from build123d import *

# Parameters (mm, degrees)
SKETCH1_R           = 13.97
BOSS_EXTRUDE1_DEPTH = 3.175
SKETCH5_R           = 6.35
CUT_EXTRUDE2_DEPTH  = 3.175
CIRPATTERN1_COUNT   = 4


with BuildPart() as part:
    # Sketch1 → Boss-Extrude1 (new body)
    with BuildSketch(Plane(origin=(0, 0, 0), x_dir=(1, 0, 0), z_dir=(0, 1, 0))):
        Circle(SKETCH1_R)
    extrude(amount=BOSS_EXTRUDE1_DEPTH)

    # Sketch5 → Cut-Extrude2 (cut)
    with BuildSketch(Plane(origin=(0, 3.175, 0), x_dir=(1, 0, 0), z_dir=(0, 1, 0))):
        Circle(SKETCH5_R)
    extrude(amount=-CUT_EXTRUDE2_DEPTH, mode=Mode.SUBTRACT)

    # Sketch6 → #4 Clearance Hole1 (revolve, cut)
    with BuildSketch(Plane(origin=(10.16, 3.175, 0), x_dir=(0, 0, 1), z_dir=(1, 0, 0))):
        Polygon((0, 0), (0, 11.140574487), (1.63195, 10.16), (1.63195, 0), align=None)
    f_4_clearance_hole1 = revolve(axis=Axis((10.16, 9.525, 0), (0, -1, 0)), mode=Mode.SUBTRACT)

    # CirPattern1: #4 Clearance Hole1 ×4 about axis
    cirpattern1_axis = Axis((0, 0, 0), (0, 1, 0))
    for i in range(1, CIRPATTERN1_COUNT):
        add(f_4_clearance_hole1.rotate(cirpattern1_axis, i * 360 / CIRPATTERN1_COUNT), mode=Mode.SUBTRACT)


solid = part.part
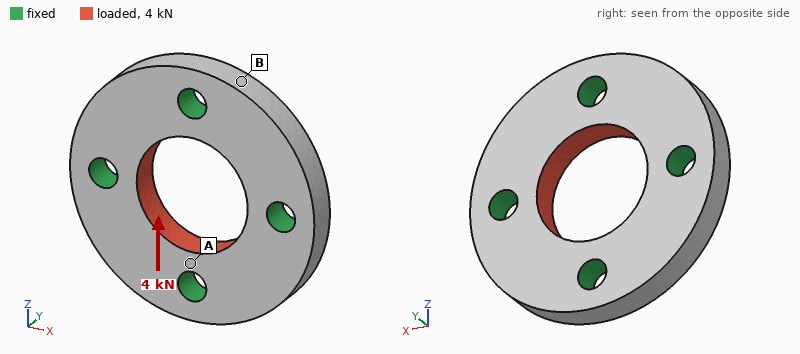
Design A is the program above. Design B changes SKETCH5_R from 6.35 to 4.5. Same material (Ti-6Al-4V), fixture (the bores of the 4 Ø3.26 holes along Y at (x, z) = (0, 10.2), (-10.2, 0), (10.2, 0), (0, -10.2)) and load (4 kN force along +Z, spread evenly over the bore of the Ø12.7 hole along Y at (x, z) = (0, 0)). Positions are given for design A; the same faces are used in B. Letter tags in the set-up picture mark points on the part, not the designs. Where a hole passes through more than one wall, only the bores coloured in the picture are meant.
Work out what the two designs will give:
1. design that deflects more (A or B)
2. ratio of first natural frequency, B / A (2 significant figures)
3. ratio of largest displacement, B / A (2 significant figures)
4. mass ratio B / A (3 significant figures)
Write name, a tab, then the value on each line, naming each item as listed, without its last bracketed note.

design that deflects more	B
ratio of first natural frequency, B / A	1.0
ratio of largest displacement, B / A	1.3
mass ratio B / A	1.14
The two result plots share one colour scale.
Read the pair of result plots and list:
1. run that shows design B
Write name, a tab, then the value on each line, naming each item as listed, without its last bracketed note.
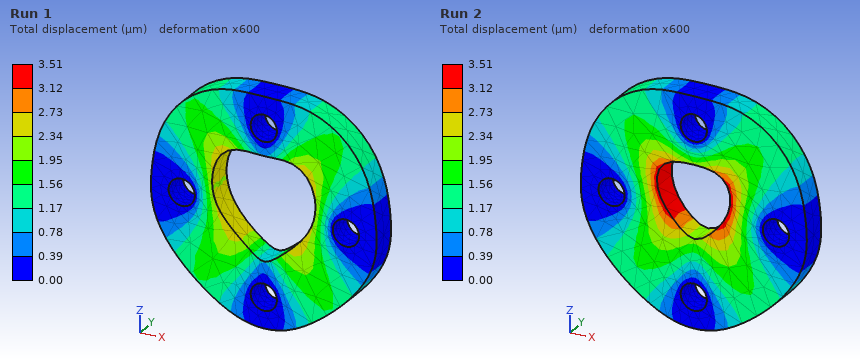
run that shows design B	Run 2
